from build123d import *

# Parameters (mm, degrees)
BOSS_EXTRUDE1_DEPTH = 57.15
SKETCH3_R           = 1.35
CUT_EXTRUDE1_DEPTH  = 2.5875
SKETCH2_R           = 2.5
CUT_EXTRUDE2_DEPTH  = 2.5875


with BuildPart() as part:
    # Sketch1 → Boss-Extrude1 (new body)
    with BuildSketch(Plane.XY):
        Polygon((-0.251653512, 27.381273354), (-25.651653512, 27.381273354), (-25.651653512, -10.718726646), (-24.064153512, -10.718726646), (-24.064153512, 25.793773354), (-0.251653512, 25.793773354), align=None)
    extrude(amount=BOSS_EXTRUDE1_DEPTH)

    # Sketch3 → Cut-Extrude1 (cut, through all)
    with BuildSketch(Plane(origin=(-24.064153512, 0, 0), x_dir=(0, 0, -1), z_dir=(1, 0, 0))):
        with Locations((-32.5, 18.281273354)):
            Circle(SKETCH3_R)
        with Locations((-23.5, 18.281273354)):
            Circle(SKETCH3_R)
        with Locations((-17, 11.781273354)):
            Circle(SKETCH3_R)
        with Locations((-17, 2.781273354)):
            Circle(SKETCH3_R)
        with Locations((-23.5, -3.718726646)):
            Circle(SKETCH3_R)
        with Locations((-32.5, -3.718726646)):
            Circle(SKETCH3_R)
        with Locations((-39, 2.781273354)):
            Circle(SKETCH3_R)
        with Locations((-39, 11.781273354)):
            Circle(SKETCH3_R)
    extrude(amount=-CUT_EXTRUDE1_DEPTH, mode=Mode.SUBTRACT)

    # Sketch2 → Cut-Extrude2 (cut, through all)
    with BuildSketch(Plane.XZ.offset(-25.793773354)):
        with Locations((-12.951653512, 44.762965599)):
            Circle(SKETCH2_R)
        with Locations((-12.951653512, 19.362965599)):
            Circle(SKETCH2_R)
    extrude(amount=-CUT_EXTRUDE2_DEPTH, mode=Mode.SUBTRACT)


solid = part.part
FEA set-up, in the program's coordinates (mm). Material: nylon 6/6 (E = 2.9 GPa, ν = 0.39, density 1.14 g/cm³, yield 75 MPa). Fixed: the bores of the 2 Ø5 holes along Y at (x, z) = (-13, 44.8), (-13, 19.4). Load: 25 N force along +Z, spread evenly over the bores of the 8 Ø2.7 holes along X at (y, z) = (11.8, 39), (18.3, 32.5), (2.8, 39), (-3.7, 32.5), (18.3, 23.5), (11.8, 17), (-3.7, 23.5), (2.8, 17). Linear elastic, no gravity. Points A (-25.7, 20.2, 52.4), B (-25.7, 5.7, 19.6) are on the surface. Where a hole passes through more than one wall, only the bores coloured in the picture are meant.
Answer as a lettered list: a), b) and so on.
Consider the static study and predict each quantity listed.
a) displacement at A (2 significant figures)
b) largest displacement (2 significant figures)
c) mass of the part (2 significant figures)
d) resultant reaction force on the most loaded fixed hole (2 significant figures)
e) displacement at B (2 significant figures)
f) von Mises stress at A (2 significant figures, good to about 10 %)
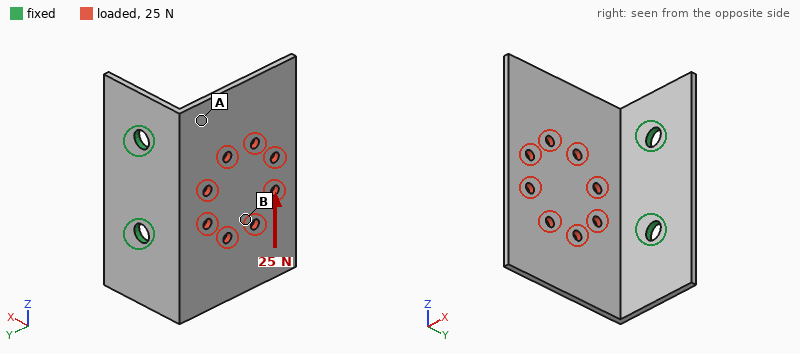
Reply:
a) 0.31 mm
b) 0.80 mm
c) 6.2 g
d) 23 N
e) 0.34 mm
f) 3.0 MPa
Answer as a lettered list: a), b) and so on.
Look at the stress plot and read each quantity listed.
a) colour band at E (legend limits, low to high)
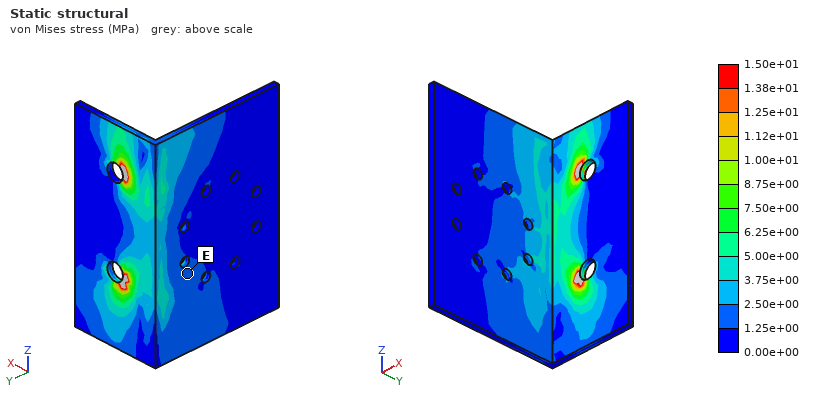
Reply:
a) 1.25e+00 to 2.50e+00 MPa
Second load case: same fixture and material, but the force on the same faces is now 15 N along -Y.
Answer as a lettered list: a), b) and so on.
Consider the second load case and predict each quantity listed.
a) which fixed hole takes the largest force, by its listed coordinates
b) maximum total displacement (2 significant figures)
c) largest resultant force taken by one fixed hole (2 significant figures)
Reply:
a) (-13, 19.4)
b) 0.67 mm
c) 9.4 N
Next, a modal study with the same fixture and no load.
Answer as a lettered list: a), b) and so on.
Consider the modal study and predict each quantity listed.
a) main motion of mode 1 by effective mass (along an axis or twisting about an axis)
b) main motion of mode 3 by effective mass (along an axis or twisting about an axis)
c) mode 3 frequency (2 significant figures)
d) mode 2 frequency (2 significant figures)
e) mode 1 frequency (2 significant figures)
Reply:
a) along X
b) along Z
c) 670 Hz
d) 410 Hz
e) 210 Hz
